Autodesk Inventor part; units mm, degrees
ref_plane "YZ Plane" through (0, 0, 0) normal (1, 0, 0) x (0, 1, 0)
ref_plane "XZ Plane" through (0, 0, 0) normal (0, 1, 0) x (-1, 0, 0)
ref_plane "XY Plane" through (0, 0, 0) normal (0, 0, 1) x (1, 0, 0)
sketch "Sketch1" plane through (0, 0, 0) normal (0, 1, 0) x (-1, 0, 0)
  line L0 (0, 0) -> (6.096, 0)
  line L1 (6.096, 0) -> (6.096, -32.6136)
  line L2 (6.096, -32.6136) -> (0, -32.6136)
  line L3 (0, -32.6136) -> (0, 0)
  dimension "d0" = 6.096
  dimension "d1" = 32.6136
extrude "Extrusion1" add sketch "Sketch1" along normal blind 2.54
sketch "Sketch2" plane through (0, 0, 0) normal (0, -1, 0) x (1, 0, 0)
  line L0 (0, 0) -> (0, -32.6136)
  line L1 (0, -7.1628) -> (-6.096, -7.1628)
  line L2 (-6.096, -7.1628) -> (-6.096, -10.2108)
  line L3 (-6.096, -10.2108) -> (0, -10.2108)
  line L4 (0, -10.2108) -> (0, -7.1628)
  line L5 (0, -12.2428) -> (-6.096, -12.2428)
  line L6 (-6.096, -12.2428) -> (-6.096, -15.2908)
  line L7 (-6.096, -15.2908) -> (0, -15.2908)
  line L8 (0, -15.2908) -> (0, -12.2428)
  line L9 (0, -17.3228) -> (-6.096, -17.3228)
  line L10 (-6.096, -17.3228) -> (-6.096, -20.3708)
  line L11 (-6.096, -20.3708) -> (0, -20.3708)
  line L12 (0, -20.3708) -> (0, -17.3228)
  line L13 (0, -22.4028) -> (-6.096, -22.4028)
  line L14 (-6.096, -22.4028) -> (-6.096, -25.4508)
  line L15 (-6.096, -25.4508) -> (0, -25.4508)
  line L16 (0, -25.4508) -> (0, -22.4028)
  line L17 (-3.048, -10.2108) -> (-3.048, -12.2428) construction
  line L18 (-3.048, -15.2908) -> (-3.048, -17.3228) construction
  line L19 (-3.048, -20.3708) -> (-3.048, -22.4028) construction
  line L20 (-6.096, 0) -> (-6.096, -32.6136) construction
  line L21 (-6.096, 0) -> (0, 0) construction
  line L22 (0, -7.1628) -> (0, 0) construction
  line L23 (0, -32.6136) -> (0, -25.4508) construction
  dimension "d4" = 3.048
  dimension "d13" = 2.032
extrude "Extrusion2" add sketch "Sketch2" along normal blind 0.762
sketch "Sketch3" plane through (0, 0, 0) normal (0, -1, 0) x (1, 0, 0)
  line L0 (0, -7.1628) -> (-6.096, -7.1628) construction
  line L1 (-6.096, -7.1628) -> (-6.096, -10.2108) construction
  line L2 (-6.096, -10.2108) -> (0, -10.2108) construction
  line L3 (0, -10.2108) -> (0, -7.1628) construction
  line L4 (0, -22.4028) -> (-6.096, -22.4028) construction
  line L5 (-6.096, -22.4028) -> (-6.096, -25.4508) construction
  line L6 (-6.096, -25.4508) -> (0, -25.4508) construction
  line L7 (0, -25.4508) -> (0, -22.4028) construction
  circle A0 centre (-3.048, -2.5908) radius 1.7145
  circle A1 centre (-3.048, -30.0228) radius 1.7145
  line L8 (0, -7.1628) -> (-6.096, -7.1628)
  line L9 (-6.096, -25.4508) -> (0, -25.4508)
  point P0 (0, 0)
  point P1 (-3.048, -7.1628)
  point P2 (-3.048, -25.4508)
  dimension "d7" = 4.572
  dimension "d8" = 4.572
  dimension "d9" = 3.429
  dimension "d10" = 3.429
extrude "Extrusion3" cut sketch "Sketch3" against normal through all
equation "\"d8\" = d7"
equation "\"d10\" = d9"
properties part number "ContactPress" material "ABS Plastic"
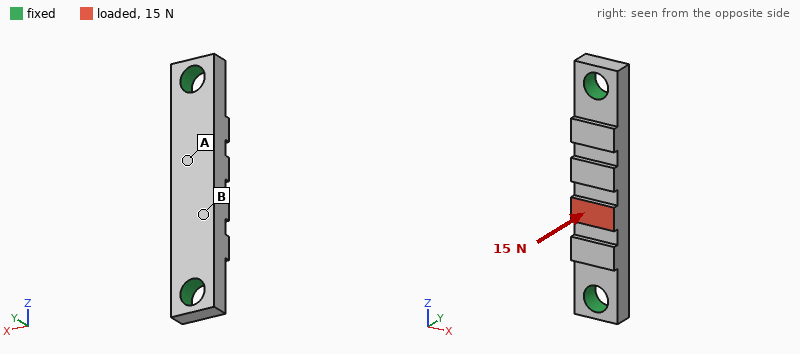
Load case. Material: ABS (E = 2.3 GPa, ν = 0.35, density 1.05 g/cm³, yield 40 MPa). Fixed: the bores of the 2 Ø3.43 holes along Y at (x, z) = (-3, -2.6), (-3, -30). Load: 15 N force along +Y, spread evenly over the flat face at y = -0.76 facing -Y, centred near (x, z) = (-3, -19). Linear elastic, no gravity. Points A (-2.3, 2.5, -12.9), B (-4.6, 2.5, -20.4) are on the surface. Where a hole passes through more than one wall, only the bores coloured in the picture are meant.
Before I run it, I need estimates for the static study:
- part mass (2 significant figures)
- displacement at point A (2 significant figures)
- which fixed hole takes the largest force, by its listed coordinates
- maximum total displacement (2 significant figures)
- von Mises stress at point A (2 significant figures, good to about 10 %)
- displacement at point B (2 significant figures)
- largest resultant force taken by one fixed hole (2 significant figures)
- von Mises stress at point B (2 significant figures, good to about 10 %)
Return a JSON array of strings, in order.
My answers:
["0.54 g", "42 µm", "(-3, -30)", "58 µm", "1.5 MPa", "48 µm", "9.8 N", "3.9 MPa"]
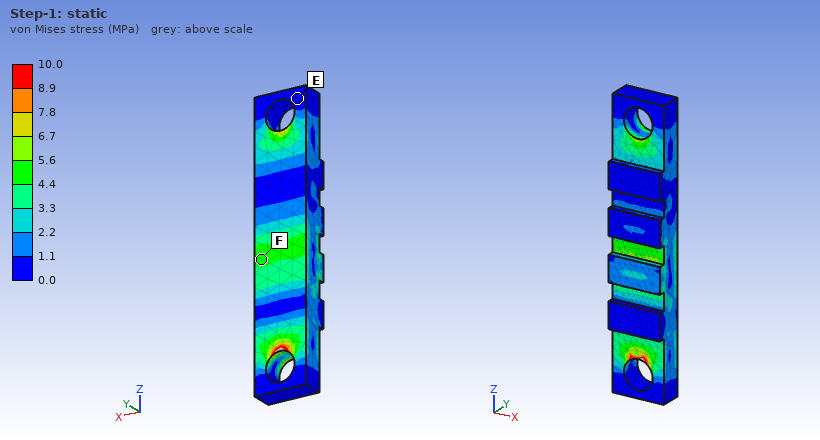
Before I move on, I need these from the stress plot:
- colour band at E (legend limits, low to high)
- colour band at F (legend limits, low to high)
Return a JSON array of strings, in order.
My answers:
["0.0 to 1.1 MPa", "4.4 to 5.6 MPa"]
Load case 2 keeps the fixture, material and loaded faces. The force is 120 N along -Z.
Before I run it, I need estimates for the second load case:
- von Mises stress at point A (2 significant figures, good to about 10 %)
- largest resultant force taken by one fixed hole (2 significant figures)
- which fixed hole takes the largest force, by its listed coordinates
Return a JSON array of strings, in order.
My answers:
["2.8 MPa", "72 N", "(-3, -30)"]
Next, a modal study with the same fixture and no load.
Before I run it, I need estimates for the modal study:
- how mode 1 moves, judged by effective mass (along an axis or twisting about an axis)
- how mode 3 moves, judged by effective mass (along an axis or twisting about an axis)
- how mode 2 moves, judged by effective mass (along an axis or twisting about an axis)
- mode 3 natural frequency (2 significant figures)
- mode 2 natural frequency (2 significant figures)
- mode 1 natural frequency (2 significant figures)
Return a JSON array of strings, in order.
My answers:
["along Y", "twisting about Z", "along X", "12 kHz", "9300 Hz", "5600 Hz"]
